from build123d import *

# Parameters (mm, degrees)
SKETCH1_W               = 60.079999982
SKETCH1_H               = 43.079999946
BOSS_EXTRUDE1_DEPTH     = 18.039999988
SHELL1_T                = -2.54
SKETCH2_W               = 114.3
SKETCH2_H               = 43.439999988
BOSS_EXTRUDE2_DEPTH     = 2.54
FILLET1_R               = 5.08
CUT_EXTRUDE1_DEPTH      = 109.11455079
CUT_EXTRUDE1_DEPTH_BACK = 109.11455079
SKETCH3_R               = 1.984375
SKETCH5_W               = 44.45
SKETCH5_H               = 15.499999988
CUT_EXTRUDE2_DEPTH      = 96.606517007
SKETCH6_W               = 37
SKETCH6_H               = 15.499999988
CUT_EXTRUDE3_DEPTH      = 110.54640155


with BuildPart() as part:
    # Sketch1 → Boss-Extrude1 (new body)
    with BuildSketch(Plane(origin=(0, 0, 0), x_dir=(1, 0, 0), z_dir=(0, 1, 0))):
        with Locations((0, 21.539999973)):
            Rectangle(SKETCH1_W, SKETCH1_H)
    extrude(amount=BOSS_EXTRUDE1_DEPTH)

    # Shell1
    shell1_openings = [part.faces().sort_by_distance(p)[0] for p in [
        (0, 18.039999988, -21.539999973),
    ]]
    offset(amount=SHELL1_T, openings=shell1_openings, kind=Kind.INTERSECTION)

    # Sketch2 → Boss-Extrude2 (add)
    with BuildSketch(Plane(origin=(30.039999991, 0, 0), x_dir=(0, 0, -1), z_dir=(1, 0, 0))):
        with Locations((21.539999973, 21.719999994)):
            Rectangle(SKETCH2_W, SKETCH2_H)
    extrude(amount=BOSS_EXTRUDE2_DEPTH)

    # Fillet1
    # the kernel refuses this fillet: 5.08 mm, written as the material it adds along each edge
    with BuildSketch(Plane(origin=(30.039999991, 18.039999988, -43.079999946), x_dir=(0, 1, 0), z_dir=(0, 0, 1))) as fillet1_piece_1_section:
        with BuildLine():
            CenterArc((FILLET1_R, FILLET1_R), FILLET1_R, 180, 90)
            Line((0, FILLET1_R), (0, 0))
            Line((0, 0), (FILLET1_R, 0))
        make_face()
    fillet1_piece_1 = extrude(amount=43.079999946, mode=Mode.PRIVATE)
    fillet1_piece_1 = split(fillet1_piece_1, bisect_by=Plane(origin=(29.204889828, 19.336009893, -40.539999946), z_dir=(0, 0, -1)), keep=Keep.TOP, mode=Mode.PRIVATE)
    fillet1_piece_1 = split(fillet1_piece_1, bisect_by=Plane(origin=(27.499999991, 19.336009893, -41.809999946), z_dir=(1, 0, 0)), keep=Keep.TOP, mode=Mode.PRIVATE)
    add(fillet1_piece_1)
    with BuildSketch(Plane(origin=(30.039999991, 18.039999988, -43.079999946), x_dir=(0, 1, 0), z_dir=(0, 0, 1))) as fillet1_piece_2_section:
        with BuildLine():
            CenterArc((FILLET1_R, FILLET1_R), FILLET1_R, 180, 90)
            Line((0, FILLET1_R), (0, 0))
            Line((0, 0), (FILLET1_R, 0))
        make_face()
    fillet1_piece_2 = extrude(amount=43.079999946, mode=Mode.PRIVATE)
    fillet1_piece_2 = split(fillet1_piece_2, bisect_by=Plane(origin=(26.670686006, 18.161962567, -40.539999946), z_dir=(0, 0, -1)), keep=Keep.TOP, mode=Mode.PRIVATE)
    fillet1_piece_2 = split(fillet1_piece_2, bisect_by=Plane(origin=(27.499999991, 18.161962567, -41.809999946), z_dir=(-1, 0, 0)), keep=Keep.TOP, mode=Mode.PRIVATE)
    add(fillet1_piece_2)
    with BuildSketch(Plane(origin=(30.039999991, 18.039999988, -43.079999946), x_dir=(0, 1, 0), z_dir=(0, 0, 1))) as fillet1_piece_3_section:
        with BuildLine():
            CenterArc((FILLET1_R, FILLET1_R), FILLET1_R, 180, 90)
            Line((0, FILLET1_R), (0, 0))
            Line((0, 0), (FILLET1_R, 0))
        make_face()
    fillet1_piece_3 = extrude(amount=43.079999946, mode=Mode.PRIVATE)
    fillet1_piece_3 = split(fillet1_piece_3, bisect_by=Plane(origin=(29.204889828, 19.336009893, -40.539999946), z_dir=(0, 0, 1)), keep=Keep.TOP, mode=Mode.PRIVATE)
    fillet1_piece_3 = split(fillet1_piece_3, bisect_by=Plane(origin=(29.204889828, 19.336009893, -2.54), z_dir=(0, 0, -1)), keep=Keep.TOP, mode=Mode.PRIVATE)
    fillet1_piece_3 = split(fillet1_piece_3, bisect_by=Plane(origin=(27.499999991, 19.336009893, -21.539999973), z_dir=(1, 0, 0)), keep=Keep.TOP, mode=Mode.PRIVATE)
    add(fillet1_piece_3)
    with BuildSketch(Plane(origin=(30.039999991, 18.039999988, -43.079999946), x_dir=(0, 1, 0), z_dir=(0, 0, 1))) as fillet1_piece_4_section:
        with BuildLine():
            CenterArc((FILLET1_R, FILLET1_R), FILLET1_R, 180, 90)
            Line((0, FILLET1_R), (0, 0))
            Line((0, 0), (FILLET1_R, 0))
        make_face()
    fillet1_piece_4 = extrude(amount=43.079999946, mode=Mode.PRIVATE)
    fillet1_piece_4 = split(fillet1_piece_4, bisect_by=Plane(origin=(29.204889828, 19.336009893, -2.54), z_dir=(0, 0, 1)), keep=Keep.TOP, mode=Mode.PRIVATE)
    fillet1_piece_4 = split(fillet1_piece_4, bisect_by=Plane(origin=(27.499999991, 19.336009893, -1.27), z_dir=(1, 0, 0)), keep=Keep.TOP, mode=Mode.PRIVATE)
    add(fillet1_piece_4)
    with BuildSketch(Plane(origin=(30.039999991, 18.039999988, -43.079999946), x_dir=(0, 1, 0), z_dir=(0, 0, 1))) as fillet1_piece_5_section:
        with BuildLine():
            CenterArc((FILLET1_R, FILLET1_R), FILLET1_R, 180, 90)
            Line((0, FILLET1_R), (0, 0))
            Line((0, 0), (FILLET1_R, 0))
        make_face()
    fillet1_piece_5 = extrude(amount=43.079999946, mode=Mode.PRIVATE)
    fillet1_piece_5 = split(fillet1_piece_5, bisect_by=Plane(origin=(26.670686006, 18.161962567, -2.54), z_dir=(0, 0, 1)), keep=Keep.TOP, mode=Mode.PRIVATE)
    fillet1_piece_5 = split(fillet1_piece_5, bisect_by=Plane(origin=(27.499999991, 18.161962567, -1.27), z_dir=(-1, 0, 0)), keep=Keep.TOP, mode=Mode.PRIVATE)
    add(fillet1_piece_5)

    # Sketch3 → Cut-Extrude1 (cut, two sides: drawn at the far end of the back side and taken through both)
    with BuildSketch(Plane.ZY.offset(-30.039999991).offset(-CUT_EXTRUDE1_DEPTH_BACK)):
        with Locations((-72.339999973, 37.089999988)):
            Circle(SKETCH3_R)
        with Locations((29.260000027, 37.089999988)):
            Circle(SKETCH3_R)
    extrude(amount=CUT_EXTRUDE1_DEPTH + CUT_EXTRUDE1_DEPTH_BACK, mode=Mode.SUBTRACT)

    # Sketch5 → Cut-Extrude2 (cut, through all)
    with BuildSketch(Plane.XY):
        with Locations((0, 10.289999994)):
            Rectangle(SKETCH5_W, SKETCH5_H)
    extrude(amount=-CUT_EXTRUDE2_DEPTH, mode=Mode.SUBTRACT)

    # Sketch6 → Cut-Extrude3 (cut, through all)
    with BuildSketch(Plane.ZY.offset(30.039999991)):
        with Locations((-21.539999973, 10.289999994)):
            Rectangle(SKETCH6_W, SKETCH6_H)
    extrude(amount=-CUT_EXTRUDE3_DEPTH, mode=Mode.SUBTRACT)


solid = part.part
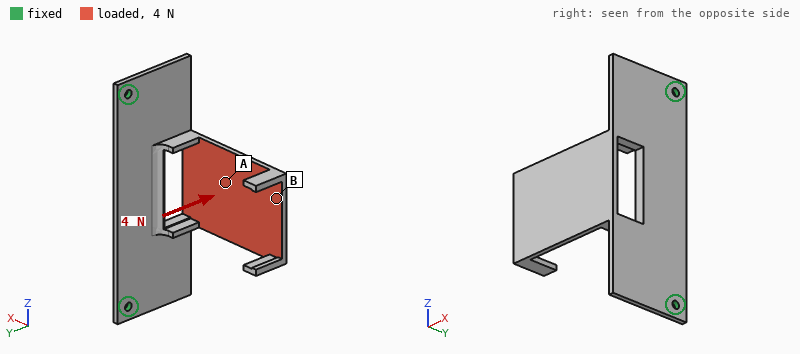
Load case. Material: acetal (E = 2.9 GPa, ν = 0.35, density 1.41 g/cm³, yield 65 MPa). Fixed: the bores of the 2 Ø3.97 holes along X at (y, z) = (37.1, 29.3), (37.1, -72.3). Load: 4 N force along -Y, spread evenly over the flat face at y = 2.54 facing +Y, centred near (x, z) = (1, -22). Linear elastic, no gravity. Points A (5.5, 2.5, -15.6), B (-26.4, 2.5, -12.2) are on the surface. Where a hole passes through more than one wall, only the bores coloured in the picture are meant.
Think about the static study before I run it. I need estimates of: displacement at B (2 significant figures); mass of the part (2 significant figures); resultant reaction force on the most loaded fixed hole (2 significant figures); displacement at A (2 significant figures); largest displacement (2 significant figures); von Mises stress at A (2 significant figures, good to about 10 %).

1.4 mm
27 g
2.8 N
0.61 mm
1.5 mm
0.98 MPa
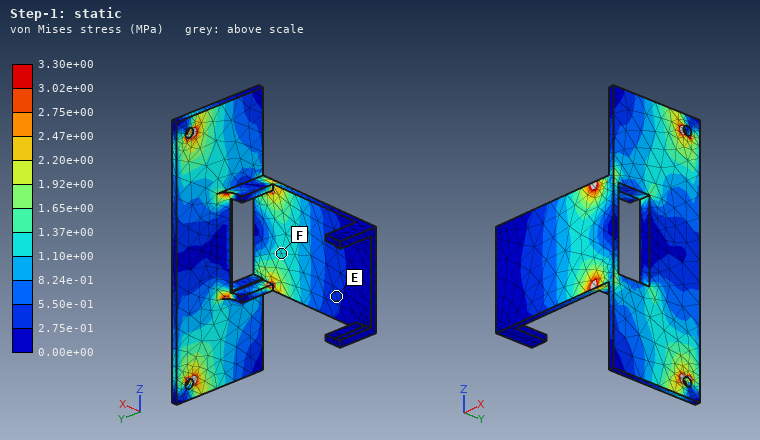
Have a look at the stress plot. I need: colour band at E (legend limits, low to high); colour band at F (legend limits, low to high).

2.75e-01 to 5.50e-01 MPa
1.10e+00 to 1.37e+00 MPa
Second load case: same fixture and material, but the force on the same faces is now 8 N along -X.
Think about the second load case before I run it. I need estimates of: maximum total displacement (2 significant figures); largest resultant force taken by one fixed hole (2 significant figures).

1.6 mm
4.0 N
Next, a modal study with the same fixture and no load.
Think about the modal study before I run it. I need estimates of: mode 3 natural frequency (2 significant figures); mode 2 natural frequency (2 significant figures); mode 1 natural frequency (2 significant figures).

190 Hz
190 Hz
84 Hz
